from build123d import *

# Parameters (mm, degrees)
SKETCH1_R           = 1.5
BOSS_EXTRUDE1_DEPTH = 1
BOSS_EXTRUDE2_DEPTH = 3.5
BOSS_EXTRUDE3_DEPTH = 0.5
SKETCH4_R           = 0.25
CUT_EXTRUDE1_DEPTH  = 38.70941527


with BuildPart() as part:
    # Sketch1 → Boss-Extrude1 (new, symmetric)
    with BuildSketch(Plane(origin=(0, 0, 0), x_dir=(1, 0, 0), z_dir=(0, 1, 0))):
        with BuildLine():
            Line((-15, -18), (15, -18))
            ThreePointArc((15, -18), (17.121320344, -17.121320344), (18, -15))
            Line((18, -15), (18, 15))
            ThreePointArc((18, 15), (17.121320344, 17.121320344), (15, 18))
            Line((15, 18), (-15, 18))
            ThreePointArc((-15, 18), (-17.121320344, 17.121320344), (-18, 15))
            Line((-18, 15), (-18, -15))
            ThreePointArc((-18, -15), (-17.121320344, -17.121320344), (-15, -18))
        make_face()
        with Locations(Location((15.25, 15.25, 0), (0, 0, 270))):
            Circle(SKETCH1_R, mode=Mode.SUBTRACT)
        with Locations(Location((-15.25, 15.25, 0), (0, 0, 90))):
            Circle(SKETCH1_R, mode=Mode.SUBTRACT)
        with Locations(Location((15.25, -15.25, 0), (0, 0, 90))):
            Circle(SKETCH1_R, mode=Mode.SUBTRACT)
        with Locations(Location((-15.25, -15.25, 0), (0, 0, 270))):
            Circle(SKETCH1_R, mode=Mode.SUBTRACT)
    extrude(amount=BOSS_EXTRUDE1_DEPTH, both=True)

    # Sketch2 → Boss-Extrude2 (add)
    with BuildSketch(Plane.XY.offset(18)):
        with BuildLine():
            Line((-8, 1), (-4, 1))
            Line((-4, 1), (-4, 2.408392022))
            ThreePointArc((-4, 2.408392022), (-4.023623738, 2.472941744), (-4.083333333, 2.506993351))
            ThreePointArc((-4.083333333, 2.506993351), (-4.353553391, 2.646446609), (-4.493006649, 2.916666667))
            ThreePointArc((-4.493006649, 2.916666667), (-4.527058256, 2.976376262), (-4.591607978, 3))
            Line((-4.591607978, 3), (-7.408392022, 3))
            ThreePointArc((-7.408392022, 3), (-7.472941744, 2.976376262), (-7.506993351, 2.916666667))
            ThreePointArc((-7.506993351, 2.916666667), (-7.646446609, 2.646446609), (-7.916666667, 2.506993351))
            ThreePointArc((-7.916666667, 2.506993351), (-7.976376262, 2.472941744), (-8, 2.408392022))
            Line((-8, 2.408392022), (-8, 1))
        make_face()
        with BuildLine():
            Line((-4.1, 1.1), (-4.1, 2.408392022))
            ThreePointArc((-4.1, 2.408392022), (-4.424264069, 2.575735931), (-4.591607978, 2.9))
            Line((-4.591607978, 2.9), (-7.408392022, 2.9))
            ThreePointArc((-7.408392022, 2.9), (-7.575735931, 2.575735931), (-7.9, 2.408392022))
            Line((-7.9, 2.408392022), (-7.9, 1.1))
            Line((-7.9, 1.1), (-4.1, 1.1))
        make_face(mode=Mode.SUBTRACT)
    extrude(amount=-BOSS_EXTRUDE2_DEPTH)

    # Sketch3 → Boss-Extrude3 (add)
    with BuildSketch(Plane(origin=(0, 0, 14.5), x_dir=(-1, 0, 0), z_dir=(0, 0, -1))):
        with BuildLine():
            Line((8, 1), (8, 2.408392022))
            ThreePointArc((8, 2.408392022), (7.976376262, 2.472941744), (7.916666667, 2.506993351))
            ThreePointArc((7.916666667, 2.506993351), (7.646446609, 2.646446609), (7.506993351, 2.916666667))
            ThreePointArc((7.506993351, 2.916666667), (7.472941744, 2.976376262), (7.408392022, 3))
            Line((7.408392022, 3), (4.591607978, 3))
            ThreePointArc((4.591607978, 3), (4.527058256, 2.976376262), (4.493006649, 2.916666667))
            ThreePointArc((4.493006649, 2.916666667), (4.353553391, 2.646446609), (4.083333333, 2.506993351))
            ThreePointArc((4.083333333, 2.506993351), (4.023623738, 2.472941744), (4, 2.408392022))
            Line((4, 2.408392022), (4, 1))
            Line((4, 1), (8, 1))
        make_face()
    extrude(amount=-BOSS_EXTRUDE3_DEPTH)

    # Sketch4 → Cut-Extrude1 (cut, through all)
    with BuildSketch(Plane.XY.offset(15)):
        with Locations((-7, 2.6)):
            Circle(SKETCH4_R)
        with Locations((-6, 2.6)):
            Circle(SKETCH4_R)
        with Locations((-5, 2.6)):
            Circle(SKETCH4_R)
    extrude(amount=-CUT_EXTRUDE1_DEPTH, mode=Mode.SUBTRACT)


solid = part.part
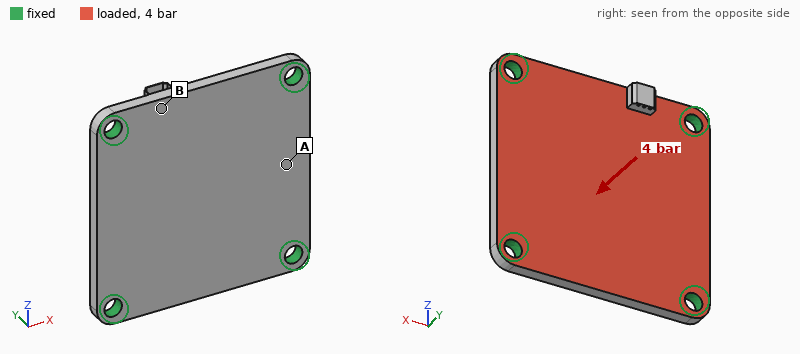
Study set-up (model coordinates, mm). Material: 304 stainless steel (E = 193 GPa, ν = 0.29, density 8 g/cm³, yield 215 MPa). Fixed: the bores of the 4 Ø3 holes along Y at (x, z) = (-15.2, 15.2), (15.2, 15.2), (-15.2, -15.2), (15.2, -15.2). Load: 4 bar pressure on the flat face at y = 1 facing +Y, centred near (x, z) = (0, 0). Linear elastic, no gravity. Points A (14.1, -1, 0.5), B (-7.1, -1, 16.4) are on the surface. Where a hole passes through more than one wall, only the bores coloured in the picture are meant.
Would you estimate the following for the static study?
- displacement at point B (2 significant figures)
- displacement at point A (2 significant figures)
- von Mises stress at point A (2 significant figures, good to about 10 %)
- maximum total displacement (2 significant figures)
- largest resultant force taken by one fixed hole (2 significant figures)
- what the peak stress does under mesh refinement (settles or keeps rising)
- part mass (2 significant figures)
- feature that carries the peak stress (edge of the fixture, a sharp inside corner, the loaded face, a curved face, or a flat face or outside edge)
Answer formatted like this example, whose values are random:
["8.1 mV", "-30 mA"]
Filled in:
["4.2 µm", "9.3 µm", "28 MPa", "16 µm", "130 N", "keeps rising", "20 g", "edge of the fixture"]
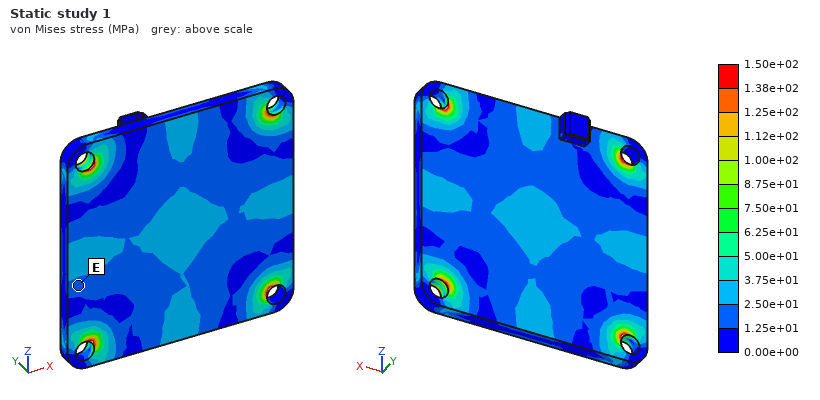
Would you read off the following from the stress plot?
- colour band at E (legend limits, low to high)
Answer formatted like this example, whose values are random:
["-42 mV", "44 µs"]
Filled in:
["1.25e+01 to 2.50e+01 MPa"]
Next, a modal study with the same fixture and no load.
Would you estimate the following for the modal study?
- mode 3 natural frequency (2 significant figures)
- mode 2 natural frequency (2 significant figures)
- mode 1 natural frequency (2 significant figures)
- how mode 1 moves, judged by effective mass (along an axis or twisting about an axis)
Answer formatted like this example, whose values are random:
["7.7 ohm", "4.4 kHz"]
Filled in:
["13 kHz", "13 kHz", "7600 Hz", "along Y"]
